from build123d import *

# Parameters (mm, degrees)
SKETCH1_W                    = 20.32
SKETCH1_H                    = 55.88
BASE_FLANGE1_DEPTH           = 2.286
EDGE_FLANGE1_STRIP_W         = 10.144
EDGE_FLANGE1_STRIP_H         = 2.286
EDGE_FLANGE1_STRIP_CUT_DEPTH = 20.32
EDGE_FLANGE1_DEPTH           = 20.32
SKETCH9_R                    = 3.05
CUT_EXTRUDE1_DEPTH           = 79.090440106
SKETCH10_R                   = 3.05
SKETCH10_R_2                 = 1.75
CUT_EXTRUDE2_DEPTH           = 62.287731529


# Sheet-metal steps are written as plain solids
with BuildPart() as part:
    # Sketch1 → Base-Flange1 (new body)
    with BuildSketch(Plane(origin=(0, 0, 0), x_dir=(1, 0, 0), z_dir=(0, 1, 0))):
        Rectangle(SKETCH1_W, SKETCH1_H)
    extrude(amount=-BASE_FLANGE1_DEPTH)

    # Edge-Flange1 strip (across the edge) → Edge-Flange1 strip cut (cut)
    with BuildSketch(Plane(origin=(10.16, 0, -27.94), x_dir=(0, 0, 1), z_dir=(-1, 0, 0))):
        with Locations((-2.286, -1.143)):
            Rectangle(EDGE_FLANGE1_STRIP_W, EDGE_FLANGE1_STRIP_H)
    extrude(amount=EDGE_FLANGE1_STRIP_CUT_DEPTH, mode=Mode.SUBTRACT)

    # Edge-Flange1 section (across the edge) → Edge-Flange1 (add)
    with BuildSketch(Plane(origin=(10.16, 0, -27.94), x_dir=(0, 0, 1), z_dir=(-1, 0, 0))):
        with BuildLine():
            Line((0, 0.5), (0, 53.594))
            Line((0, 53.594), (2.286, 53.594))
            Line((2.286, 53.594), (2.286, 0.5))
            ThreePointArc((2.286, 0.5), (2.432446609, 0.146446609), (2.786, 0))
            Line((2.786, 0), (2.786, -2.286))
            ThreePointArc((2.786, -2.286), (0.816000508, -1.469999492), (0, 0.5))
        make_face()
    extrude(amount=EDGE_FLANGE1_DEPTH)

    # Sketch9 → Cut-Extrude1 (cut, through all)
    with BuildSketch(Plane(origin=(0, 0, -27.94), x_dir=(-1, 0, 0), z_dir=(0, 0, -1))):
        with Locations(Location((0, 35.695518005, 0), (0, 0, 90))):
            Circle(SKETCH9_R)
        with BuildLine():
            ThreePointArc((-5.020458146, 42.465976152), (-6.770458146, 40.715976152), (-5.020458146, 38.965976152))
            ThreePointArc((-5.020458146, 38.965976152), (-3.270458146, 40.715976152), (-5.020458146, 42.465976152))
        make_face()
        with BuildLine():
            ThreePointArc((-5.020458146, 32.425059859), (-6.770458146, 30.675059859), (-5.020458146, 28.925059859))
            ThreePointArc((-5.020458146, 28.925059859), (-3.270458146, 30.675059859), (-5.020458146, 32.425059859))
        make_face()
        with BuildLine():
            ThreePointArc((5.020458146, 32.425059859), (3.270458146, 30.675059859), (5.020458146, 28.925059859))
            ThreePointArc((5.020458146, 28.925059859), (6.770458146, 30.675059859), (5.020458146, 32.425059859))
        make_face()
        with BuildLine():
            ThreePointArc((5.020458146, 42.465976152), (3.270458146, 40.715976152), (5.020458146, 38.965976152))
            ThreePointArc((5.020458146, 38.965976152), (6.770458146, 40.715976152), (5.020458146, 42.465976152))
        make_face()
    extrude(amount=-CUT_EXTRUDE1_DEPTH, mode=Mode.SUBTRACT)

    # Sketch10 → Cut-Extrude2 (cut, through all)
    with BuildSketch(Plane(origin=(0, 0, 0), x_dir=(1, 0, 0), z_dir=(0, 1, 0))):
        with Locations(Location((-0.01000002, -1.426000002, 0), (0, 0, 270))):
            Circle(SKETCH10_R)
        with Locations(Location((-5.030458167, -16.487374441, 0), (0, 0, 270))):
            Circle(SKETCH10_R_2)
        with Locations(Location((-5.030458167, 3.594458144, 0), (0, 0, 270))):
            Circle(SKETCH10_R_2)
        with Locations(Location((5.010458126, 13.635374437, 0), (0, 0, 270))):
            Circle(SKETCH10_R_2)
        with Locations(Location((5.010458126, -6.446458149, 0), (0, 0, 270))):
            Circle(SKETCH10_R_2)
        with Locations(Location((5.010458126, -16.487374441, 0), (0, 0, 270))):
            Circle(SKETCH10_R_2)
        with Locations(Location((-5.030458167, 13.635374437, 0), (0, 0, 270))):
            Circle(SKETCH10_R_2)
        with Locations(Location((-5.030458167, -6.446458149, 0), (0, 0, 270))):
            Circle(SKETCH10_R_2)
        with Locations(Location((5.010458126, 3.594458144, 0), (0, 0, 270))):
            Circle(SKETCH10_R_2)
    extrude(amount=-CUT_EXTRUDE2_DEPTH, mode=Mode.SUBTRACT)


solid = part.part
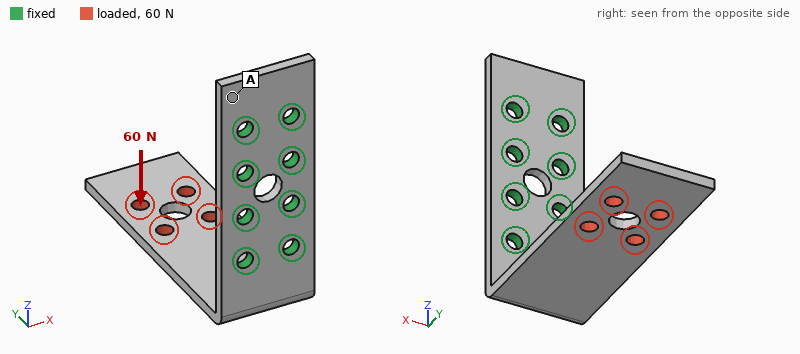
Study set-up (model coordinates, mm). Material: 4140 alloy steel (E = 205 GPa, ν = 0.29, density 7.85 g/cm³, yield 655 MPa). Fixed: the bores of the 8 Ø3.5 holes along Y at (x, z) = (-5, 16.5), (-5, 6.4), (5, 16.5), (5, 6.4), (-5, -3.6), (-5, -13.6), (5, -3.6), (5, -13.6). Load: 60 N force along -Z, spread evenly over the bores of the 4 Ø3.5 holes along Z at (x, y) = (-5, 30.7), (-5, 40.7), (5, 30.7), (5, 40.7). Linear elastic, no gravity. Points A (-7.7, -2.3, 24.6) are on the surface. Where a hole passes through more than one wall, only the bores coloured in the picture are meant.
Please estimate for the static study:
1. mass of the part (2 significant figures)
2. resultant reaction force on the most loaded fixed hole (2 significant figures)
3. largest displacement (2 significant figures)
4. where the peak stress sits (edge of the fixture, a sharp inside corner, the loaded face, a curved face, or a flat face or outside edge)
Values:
37 g
36 N
0.74 mm
a curved face
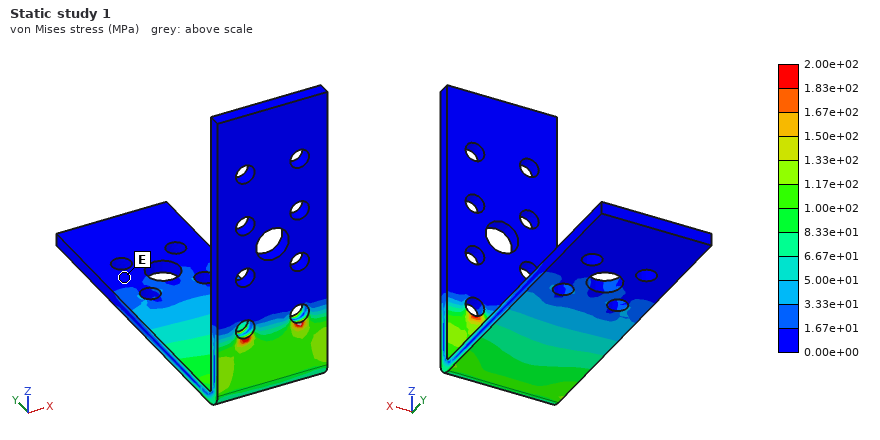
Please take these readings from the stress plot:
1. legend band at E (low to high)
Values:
0.00e+00 to 1.67e+01 MPa
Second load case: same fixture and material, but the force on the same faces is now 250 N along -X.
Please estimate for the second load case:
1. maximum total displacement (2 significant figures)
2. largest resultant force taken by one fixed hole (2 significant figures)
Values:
0.56 mm
760 N
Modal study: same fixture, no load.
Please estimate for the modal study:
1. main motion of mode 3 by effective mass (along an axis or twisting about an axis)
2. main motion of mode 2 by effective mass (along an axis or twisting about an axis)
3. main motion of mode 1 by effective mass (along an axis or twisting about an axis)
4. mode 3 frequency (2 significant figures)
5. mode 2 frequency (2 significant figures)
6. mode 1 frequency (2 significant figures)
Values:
along Y
along X
along Z
2700 Hz
1100 Hz
490 Hz
